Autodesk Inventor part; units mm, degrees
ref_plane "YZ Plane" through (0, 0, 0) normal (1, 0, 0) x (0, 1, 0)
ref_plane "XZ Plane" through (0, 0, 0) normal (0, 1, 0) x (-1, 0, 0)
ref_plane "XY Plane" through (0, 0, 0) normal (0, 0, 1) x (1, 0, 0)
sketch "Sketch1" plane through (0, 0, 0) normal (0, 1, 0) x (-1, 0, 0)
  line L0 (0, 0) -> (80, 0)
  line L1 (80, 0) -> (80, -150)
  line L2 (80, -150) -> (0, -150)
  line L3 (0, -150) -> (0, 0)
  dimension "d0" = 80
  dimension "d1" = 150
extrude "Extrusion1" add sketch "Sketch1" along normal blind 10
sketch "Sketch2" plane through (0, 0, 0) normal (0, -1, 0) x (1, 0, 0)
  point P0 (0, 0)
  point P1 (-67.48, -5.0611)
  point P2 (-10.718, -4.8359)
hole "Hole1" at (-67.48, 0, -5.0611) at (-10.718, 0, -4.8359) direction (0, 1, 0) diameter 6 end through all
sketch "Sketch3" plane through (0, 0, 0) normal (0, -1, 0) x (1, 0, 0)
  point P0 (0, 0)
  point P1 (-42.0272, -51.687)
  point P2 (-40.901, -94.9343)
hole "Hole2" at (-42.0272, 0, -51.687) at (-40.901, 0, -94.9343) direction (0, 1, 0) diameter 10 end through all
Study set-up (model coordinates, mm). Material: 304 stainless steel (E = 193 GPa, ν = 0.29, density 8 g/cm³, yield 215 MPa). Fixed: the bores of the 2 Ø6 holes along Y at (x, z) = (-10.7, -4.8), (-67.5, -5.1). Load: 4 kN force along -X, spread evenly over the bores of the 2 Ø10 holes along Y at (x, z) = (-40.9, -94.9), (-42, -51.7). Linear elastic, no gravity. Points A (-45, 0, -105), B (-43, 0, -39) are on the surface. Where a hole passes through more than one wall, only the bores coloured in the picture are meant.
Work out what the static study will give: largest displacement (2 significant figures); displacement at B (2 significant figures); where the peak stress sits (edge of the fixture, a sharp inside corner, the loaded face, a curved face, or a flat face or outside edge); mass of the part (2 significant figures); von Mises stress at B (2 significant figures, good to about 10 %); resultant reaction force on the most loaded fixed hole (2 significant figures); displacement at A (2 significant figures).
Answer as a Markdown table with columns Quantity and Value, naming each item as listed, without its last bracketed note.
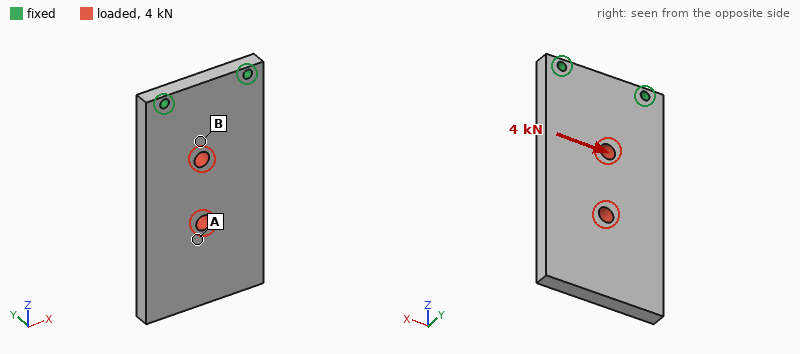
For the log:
| Quantity | Value |
|---|---|
| largest displacement | 25 µm |
| displacement at B | 5.5 µm |
| where the peak stress sits | edge of the fixture |
| mass of the part | 940 g |
| von Mises stress at B | 16 MPa |
| resultant reaction force on the most loaded fixed hole | 5.0 kN |
| displacement at A | 18 µm |
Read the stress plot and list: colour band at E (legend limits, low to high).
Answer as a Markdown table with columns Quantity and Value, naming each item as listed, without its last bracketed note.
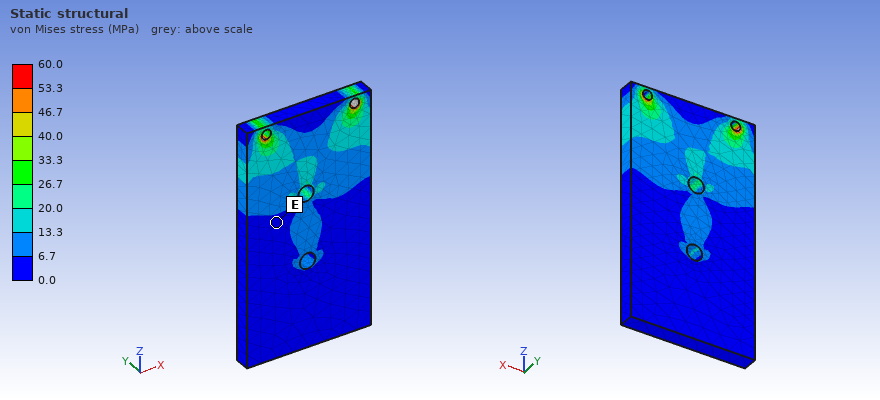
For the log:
| Quantity | Value |
|---|---|
| colour band at E | 0.0 to 6.7 MPa |
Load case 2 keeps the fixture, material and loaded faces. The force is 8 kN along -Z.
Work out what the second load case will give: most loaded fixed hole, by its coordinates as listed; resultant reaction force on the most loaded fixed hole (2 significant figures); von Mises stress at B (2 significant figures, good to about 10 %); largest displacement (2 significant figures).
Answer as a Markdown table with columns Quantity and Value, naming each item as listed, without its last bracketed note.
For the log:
| Quantity | Value |
|---|---|
| most loaded fixed hole, by its coordinates as listed | (-67.5, -5.1) |
| resultant reaction force on the most loaded fixed hole | 4.4 kN |
| von Mises stress at B | 12 MPa |
| largest displacement | 5.8 µm |
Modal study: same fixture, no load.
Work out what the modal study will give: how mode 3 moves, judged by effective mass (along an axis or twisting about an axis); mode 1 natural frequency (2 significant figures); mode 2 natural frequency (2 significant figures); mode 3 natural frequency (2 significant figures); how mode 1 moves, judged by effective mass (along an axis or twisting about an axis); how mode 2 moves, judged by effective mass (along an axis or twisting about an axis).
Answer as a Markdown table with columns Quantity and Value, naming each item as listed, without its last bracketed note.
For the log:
| Quantity | Value |
|---|---|
| how mode 3 moves, judged by effective mass | along Y |
| mode 1 natural frequency | 340 Hz |
| mode 2 natural frequency | 1400 Hz |
| mode 3 natural frequency | 2200 Hz |
| how mode 1 moves, judged by effective mass | along Y |
| how mode 2 moves, judged by effective mass | twisting about Z |
